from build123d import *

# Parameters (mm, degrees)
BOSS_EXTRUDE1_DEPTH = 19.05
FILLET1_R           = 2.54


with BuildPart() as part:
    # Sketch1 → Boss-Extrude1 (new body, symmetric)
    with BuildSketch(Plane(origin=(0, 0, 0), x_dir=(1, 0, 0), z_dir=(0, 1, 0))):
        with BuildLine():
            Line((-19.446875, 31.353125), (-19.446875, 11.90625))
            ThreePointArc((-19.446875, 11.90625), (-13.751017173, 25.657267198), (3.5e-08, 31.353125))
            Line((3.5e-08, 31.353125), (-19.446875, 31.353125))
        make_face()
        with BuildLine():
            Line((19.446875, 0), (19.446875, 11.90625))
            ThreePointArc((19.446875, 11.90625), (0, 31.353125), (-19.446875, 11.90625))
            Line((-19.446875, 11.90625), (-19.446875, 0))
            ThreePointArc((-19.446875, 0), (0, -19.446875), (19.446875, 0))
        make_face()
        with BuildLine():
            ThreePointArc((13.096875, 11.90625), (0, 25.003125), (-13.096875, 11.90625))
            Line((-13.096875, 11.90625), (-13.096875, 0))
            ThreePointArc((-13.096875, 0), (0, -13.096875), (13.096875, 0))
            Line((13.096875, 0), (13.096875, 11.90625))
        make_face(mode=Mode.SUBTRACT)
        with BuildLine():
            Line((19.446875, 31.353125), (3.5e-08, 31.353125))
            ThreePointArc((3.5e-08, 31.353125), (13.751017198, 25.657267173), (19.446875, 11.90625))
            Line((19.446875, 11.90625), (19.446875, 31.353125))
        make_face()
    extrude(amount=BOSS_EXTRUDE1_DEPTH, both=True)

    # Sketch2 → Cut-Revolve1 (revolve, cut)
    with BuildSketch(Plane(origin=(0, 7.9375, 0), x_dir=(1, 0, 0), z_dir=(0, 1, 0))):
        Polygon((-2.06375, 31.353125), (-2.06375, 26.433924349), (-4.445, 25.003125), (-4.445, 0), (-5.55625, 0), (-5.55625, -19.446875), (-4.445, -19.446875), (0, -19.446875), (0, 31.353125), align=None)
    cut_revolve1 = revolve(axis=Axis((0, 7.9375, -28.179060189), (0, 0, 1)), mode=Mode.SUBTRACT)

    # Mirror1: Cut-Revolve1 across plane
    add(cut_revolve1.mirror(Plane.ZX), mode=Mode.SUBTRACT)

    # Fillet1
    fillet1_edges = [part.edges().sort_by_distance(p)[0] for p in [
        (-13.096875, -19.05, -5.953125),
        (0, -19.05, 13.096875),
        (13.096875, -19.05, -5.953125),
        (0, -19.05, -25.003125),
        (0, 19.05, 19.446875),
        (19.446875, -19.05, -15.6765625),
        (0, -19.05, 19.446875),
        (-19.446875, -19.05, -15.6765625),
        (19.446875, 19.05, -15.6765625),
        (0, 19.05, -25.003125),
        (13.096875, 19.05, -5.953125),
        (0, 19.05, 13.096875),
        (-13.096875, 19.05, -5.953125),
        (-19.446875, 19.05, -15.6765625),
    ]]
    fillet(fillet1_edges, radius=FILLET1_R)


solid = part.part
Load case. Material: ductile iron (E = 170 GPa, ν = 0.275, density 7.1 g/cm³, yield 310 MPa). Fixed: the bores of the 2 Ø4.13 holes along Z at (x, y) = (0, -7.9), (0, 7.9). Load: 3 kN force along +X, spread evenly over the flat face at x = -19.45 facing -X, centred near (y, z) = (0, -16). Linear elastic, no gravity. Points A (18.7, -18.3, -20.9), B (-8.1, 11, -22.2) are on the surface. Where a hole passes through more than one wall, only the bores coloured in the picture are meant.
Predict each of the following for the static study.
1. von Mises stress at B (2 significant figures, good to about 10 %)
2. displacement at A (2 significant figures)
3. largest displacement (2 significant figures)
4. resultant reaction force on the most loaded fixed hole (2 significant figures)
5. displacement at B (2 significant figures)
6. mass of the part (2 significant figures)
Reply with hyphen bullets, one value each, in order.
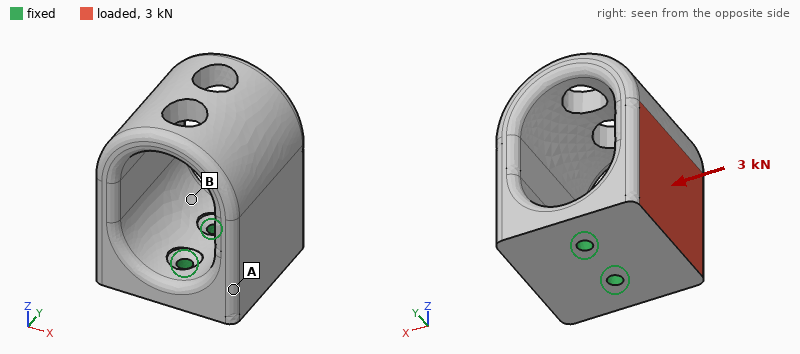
- 40 MPa
- 26 µm
- 84 µm
- 1.5 kN
- 17 µm
- 250 g
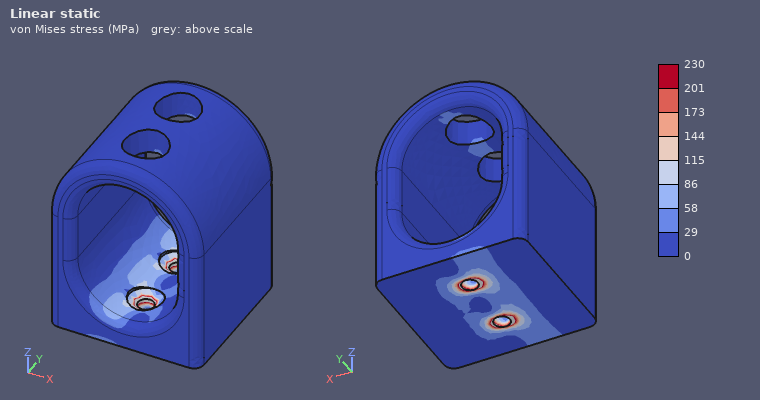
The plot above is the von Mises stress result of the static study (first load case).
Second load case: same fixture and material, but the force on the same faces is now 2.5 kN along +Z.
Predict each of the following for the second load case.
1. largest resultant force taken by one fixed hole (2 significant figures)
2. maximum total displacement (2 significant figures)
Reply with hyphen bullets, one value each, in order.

- 1.3 kN
- 90 µm
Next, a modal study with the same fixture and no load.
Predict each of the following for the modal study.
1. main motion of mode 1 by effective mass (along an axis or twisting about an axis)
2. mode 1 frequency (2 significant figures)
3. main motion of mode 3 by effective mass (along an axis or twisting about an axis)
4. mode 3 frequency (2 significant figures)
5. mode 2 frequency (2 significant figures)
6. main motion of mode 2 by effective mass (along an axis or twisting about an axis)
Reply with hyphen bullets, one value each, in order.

- along X
- 1800 Hz
- along Z
- 5900 Hz
- 3500 Hz
- along Y
